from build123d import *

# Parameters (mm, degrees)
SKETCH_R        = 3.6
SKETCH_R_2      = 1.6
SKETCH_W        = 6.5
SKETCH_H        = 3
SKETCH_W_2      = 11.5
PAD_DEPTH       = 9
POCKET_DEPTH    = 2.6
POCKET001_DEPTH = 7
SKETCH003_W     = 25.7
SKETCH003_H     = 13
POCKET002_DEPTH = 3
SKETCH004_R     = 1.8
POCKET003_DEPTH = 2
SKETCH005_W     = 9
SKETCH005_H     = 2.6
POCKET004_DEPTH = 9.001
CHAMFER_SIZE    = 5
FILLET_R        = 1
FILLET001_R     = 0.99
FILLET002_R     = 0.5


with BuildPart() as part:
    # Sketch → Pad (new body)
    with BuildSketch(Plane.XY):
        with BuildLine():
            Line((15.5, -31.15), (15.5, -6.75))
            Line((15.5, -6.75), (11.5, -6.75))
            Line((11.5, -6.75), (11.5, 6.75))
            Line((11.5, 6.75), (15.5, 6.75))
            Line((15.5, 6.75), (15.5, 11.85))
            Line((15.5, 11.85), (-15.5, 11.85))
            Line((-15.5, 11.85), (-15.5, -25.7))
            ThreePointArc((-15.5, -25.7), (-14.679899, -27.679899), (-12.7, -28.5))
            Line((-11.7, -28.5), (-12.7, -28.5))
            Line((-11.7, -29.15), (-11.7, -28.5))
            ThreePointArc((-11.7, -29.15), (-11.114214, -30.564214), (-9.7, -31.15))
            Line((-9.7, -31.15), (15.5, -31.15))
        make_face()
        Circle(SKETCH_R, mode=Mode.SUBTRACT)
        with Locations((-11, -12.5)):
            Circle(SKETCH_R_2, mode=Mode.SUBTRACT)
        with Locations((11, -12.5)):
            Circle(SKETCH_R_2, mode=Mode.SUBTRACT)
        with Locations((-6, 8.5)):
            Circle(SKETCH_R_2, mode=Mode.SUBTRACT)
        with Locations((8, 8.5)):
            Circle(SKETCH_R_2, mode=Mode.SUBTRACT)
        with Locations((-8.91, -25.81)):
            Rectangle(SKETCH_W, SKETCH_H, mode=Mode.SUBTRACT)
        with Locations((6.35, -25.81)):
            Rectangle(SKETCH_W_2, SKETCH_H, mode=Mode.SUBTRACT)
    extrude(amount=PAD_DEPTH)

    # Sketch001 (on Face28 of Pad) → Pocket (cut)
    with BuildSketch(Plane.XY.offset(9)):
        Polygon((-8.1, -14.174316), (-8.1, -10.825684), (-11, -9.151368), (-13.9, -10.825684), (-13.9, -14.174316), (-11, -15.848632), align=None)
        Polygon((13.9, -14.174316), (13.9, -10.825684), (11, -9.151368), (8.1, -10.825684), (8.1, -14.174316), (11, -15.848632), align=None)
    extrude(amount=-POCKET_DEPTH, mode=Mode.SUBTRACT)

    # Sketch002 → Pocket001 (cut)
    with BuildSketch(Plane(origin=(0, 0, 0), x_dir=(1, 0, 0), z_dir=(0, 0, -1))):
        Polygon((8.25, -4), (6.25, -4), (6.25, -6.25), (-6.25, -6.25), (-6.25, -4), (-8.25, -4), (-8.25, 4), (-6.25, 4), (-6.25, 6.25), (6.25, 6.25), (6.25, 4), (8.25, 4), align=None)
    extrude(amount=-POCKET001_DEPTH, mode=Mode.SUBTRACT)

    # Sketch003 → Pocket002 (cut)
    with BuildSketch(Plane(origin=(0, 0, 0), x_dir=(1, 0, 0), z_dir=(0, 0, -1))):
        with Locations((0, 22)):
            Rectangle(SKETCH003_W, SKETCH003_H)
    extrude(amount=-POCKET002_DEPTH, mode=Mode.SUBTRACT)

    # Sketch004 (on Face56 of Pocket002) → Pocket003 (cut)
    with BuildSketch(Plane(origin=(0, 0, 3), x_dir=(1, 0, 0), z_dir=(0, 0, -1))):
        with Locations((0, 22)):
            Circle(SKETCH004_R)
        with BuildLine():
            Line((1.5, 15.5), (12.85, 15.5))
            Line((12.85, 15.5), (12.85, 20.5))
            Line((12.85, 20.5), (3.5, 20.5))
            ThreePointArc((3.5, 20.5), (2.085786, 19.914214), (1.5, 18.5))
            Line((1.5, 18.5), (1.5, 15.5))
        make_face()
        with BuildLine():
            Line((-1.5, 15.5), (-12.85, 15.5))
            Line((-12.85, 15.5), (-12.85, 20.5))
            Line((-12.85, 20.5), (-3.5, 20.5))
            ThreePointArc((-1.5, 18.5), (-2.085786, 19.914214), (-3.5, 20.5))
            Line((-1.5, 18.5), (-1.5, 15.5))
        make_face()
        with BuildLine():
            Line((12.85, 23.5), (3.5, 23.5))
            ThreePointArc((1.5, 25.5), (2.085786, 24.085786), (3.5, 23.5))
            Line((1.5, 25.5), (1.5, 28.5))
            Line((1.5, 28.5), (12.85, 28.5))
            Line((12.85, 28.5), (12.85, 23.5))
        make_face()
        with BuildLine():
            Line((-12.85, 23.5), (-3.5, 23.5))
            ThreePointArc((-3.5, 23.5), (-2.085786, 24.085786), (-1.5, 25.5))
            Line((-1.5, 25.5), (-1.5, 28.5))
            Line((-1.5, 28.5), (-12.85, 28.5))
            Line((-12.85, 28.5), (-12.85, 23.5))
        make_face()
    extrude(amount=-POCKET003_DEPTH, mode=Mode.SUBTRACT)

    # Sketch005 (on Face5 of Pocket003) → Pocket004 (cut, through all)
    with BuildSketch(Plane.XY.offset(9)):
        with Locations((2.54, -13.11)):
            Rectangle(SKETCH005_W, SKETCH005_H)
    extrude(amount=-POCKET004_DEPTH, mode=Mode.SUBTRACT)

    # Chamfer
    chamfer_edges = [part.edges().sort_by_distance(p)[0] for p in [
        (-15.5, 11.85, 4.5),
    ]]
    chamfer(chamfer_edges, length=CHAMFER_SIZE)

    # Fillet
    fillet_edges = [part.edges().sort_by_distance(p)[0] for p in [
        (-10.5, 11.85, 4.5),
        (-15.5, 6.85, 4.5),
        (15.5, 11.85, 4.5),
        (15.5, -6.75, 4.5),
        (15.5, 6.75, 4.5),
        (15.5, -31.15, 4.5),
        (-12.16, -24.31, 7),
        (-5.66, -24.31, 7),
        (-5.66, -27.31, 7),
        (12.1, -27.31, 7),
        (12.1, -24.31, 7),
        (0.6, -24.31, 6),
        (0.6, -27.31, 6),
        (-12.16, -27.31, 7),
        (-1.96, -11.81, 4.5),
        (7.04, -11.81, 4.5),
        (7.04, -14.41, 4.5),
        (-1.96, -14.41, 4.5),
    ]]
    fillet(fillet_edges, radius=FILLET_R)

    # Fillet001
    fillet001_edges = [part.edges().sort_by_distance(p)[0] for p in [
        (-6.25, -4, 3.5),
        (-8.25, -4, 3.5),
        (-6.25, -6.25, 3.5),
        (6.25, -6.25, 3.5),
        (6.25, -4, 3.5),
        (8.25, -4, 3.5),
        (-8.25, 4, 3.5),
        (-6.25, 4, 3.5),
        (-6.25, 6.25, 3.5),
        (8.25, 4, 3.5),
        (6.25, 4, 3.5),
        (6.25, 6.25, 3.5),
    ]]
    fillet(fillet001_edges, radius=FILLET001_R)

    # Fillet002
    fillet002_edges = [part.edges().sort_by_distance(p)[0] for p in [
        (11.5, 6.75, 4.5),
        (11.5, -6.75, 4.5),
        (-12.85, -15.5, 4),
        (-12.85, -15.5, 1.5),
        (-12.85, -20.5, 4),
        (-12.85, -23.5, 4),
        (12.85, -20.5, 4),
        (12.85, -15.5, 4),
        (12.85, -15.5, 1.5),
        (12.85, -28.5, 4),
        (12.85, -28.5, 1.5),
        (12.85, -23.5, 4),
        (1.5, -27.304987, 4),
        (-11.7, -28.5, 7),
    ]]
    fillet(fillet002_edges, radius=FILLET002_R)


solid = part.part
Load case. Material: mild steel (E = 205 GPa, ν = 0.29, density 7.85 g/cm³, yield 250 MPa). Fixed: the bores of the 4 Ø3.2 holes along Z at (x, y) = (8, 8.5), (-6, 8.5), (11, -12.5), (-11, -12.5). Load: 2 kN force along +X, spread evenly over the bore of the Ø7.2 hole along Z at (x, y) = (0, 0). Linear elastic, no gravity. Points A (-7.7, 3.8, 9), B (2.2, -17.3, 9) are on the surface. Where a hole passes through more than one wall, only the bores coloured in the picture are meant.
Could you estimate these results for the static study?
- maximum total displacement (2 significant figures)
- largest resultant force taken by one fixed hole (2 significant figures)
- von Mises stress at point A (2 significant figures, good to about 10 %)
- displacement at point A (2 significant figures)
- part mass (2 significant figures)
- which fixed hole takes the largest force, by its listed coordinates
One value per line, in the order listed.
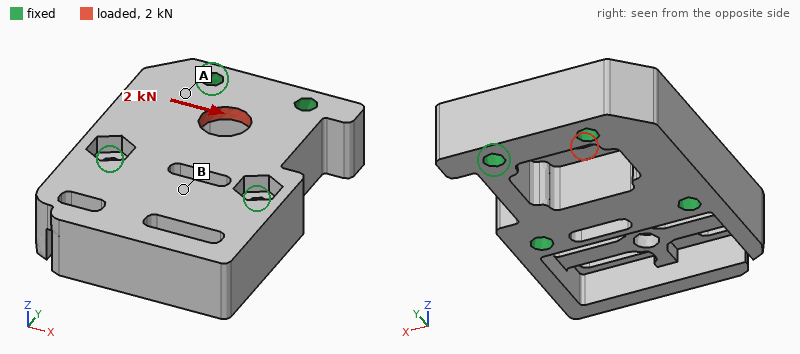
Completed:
2.2 µm
630 N
25 MPa
0.85 µm
60 g
(-6, 8.5)
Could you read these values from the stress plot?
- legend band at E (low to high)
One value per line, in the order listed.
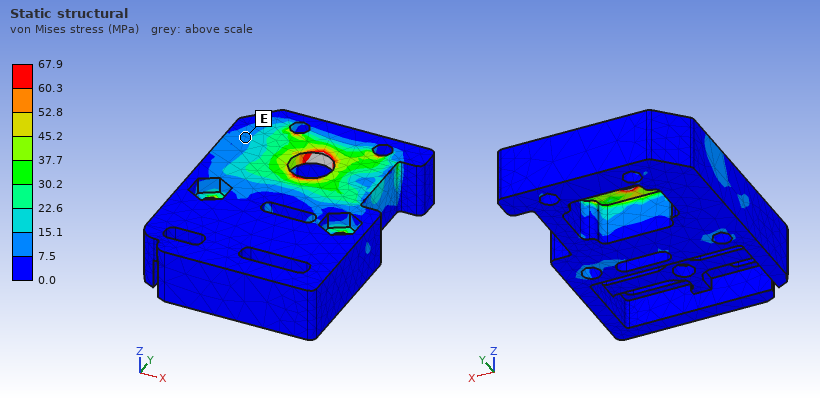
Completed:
7.5 to 15.1 MPa
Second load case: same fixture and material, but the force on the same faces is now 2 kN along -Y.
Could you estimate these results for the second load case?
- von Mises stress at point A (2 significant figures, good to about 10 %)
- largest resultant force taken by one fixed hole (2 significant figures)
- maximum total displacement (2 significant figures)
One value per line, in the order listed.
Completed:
12 MPa
690 N
2.4 µm
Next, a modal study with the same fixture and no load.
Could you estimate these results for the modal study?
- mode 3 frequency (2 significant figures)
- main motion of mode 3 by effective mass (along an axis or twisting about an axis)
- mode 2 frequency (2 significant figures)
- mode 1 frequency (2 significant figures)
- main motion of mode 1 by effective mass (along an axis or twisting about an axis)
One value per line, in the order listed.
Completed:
26 kHz
along X
16 kHz
10 kHz
along Z
